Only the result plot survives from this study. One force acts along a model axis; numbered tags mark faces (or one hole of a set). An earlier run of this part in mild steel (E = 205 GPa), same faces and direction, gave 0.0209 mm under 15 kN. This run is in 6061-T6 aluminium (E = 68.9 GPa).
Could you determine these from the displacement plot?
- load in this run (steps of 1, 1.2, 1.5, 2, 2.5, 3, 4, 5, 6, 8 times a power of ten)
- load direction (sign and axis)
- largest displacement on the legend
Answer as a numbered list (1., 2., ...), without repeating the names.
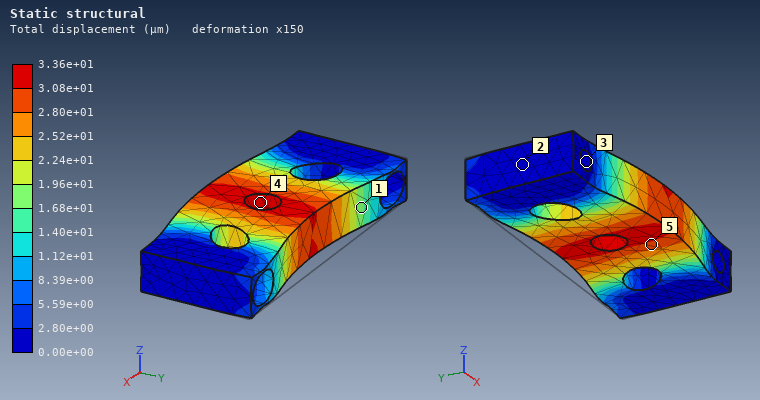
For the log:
1. 8 kN
2. -Y
3. 3.36e+01 µm
